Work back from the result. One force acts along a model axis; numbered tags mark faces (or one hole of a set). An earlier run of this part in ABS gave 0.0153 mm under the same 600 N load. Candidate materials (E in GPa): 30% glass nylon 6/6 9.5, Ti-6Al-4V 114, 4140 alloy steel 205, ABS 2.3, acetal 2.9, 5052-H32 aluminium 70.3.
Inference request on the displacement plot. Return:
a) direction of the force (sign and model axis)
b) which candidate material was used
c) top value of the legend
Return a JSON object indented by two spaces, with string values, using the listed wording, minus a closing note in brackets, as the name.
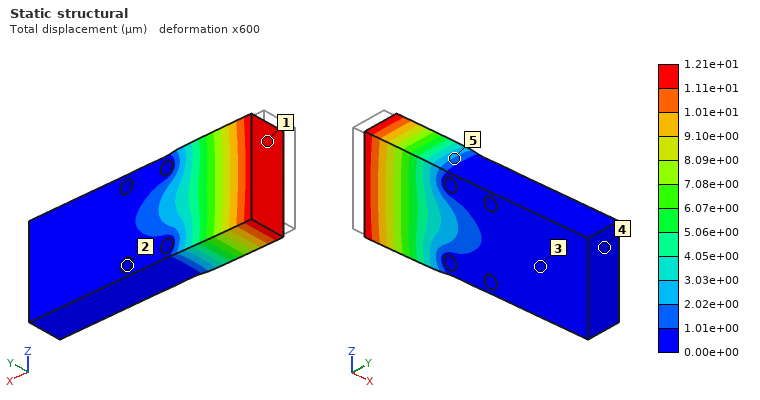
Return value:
{
  "direction of the force": "+X",
  "which candidate material was used": "acetal",
  "top value of the legend": "1.21e+01 µm"
}
